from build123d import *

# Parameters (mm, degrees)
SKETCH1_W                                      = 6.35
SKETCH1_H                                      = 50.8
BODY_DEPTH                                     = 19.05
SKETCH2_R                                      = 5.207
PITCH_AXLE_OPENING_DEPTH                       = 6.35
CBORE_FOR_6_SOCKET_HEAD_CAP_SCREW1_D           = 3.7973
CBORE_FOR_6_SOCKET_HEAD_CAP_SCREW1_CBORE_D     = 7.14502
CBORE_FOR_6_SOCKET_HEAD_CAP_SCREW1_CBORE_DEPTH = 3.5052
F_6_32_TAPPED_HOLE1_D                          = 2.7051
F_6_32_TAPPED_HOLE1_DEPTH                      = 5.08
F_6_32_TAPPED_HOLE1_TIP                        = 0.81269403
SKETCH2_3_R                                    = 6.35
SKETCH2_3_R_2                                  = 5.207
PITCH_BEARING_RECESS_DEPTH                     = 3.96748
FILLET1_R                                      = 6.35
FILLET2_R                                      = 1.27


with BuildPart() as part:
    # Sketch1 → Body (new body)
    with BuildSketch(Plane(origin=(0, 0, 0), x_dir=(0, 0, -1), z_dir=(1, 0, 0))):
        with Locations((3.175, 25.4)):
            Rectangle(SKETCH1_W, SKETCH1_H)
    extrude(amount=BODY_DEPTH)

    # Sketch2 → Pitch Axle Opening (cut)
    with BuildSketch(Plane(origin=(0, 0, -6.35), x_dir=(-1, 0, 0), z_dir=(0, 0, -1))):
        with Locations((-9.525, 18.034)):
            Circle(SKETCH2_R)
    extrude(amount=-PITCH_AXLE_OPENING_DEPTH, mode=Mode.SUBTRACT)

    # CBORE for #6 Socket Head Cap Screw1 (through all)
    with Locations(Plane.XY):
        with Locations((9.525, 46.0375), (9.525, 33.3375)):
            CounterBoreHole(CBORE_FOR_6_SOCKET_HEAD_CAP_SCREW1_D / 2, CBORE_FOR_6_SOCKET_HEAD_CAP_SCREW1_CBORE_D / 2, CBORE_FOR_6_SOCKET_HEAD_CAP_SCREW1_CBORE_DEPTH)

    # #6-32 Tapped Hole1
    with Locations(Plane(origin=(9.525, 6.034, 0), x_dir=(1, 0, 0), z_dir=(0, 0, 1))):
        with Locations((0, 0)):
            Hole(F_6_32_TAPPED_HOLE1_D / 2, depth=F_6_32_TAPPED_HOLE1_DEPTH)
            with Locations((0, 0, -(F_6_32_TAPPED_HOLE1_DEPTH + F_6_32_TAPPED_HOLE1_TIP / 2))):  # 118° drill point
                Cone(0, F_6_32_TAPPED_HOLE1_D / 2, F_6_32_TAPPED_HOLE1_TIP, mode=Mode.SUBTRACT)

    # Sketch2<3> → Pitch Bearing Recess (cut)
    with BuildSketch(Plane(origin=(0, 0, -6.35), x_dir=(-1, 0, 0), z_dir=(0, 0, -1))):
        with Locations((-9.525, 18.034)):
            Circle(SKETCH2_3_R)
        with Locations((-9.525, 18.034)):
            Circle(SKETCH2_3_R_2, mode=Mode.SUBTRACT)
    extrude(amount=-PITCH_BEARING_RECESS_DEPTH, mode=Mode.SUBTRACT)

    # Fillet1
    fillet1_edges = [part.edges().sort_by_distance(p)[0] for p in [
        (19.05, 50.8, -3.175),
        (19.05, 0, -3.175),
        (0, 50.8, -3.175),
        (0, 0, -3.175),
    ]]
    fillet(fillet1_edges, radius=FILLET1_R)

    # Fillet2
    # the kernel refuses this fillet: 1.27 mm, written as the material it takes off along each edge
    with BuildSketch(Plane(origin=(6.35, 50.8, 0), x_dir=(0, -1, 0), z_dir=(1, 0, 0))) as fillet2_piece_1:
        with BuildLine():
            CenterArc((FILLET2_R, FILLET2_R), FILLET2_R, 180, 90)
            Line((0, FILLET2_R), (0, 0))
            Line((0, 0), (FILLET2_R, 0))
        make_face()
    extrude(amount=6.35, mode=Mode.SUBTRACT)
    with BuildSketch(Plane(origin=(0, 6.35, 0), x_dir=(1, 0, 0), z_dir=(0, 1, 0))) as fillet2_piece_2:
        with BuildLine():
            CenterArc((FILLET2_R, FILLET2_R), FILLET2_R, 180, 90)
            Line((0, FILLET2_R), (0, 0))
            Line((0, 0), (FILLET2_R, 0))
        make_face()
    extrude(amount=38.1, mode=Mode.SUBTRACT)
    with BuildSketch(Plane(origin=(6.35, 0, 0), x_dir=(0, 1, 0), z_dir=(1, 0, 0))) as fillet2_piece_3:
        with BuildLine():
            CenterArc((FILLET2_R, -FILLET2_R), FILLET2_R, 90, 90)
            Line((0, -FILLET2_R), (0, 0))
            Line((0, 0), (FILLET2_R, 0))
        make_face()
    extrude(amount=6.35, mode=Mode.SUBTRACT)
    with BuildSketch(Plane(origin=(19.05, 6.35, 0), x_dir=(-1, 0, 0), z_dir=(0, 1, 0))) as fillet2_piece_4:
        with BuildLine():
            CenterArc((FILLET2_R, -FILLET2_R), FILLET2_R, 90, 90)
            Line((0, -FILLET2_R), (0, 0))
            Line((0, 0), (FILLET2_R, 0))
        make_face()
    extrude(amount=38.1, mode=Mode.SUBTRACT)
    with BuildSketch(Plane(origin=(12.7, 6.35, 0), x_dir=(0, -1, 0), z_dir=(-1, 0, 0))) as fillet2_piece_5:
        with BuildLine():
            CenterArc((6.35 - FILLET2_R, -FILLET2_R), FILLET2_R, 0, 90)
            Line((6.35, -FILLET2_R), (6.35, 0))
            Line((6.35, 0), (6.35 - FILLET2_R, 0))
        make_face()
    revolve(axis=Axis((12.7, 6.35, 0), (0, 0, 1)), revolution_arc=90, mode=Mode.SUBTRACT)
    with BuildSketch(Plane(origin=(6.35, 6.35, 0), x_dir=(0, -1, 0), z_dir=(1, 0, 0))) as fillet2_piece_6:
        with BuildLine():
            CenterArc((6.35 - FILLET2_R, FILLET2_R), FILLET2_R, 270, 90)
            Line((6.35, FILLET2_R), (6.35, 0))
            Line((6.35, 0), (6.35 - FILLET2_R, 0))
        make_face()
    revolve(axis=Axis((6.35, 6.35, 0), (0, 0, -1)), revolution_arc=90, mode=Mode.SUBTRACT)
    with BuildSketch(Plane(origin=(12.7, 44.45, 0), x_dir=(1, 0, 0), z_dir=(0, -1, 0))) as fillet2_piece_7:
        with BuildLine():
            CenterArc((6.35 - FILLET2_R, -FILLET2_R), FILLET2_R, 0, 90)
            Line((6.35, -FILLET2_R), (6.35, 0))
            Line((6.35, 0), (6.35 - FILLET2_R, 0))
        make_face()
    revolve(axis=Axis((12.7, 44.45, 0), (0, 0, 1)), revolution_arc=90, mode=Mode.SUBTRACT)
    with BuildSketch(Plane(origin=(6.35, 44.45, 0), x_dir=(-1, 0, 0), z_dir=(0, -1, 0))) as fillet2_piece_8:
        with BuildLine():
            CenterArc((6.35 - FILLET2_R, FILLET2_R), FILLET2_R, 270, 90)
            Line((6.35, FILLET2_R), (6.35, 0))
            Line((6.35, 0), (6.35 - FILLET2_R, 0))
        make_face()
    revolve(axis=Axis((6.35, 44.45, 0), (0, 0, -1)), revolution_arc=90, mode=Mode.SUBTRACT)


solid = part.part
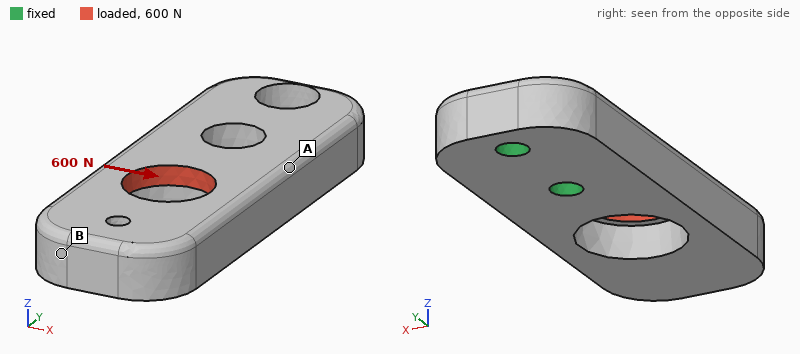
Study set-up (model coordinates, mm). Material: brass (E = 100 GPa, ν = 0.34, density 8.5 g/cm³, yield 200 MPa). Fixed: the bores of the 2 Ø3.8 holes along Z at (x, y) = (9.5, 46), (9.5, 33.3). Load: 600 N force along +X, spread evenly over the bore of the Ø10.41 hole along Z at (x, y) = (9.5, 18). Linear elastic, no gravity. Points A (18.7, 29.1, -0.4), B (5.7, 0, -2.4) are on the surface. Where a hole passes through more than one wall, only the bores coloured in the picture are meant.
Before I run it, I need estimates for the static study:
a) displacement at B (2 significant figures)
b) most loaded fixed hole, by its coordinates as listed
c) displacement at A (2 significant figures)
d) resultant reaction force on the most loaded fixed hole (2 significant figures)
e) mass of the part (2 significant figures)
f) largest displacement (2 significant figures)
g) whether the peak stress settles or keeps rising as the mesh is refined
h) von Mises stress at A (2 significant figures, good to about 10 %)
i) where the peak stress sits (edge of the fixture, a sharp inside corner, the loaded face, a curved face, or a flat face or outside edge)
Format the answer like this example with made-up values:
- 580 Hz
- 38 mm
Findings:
- 29 µm
- (9.5, 33.3)
- 9.6 µm
- 1.1 kN
- 41 g
- 31 µm
- keeps rising
- 22 MPa
- edge of the fixture
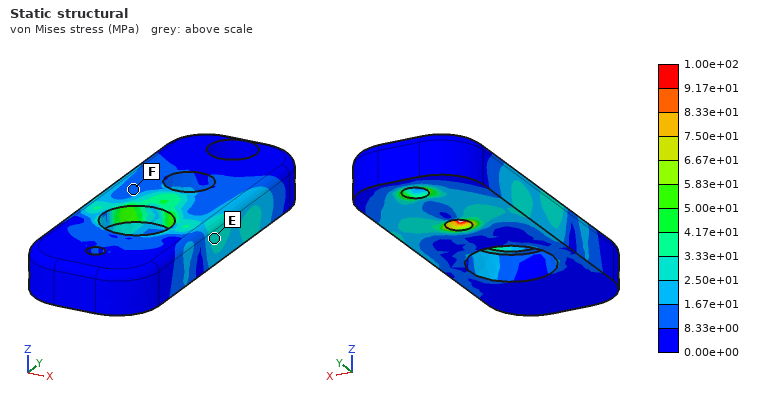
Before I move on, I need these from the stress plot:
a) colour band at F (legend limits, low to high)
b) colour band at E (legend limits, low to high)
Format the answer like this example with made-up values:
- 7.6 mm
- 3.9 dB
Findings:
- 8.33e+00 to 1.67e+01 MPa
- 2.50e+01 to 3.33e+01 MPa
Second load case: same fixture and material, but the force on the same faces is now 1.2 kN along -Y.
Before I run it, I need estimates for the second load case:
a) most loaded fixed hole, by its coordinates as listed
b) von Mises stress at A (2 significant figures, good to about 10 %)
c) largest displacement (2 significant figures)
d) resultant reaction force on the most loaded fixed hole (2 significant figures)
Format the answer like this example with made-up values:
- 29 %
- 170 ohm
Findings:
- (9.5, 33.3)
- 36 MPa
- 50 µm
- 730 N
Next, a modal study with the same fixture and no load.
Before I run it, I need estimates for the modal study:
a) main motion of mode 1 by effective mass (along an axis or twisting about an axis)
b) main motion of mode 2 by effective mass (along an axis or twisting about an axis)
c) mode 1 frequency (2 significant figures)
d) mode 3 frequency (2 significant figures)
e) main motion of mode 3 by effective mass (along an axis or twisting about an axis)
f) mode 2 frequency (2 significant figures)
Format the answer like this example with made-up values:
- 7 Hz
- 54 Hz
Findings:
- along Z
- along X
- 2400 Hz
- 6300 Hz
- twisting about Y
- 4900 Hz
